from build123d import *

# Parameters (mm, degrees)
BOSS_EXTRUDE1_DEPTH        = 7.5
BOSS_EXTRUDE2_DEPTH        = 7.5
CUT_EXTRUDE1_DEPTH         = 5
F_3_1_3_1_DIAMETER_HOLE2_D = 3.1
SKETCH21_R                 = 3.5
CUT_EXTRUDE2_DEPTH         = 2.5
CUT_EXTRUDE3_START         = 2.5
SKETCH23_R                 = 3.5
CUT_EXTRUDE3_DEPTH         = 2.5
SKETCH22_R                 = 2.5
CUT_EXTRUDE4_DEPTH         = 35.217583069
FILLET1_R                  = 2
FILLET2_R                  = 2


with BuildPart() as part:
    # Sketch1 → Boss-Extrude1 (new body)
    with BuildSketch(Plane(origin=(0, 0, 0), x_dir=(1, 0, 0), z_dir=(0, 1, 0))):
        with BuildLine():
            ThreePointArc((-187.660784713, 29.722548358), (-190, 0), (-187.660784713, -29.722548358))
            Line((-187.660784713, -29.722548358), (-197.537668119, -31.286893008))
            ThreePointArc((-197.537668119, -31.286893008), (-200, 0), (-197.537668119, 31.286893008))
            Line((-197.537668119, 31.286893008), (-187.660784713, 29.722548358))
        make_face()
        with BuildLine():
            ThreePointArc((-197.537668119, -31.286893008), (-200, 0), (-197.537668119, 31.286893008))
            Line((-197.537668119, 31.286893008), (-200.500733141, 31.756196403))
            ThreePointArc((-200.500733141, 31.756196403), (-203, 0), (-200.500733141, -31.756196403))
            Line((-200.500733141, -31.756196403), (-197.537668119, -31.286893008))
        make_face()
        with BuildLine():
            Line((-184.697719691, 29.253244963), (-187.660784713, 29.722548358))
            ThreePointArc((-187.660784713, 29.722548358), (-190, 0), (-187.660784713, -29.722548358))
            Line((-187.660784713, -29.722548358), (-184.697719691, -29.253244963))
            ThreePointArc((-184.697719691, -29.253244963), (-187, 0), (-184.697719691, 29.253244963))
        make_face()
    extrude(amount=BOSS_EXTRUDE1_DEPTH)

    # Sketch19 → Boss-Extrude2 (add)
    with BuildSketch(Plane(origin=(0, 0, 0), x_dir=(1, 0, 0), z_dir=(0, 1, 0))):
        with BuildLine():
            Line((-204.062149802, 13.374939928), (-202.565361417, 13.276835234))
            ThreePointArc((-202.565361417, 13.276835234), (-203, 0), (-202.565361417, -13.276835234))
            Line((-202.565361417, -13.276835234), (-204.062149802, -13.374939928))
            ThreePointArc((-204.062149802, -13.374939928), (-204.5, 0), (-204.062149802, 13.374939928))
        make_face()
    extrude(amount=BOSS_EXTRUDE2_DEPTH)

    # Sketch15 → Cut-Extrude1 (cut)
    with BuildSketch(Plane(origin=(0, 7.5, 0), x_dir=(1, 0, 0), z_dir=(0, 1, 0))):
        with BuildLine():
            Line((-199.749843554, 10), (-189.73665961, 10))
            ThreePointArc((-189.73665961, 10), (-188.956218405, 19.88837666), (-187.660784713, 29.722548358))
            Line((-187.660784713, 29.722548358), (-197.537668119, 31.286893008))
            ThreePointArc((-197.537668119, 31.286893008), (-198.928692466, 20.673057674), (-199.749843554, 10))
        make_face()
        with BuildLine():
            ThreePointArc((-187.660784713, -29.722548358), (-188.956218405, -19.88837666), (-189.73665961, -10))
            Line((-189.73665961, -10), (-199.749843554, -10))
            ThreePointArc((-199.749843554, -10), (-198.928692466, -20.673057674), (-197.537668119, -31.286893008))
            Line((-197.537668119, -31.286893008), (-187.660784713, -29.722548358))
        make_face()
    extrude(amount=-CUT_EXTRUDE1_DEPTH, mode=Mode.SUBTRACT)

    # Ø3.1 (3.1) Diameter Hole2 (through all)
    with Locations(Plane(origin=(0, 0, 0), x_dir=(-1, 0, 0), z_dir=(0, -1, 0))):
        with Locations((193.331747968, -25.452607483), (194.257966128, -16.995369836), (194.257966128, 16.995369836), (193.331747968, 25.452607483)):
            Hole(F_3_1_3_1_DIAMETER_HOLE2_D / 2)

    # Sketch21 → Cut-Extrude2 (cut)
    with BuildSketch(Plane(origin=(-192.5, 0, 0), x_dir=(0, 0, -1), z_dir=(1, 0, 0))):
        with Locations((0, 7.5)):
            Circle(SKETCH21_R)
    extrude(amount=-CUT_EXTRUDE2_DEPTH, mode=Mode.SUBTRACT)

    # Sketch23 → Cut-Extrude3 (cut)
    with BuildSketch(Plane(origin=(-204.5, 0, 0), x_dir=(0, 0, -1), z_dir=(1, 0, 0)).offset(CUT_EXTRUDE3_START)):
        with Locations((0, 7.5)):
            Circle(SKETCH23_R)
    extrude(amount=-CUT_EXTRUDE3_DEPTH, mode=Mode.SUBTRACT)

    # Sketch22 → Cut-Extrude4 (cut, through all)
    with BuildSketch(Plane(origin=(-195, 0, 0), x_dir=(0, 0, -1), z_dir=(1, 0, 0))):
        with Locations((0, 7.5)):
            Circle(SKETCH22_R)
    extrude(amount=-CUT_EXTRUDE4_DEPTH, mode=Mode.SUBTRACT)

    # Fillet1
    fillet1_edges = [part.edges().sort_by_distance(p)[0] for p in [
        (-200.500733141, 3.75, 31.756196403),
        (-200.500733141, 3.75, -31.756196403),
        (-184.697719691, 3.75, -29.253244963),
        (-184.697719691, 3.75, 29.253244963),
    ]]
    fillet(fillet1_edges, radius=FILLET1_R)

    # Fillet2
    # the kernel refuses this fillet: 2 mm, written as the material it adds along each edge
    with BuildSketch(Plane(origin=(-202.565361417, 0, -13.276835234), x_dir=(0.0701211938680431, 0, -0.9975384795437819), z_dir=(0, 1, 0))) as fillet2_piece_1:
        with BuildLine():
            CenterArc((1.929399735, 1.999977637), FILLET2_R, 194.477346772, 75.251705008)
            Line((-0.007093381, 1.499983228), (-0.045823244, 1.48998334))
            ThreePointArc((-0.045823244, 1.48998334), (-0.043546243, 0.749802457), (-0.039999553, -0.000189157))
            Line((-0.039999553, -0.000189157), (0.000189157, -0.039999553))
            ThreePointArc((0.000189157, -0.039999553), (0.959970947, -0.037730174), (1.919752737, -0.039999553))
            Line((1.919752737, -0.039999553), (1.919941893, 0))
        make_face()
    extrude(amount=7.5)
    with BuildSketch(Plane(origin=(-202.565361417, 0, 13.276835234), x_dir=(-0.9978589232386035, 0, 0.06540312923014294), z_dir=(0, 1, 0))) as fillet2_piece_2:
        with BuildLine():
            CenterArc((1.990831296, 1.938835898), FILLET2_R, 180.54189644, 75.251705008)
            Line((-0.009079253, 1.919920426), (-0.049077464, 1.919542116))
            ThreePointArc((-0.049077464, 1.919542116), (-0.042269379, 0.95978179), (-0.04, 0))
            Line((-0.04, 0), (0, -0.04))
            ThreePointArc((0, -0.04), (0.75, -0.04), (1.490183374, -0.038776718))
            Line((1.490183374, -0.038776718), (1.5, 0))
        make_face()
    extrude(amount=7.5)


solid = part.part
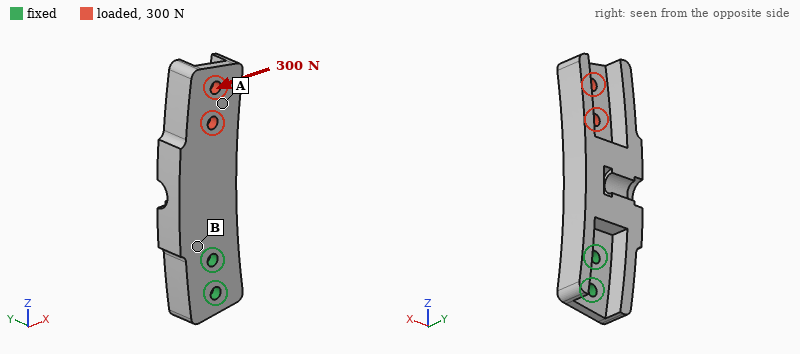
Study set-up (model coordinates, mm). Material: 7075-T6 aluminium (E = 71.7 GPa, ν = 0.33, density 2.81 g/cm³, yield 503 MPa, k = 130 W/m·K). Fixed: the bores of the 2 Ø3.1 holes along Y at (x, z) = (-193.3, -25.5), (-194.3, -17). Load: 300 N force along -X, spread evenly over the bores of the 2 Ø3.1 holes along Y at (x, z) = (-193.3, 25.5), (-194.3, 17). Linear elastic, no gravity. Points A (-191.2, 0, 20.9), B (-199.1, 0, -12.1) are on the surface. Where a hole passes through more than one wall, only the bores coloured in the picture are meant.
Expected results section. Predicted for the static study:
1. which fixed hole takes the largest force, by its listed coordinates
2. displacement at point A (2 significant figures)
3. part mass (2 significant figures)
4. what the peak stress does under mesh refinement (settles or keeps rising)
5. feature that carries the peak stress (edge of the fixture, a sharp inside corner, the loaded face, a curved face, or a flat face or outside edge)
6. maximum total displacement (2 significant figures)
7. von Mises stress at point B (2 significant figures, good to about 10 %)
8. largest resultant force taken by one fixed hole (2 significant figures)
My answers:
(-194.3, -17)
0.094 mm
15 g
keeps rising
edge of the fixture
0.12 mm
32 MPa
1.2 kN
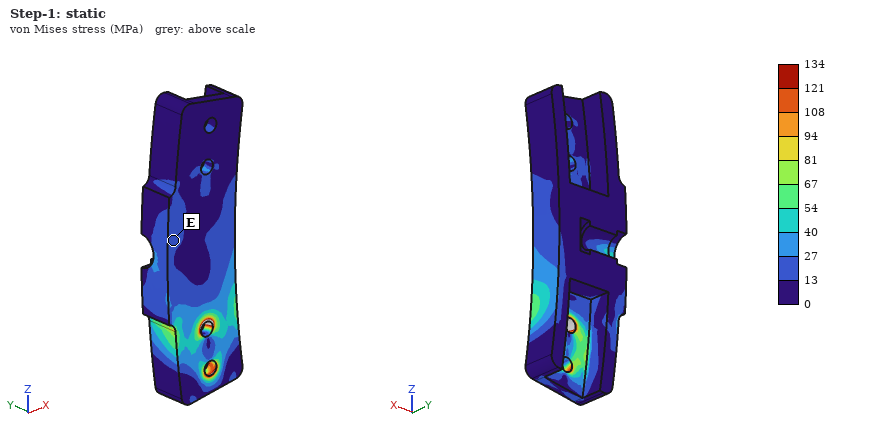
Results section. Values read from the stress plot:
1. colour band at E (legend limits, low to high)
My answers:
13 to 27 MPa
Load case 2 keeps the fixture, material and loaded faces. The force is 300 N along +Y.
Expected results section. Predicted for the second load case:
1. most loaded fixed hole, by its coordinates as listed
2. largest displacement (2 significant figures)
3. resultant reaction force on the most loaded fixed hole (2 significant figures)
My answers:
(-194.3, -17)
0.51 mm
1.2 kN
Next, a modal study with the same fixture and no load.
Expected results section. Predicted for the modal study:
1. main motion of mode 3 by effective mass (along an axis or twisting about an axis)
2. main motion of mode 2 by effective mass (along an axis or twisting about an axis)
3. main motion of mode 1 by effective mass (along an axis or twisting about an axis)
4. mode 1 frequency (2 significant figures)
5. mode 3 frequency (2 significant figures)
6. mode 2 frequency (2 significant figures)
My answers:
twisting about Z
along X
along Y
2000 Hz
5800 Hz
3900 Hz
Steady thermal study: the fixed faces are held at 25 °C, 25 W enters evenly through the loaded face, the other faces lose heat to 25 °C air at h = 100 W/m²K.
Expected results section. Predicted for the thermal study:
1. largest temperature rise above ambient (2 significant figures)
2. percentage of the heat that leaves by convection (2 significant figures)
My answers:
72 K
43 %
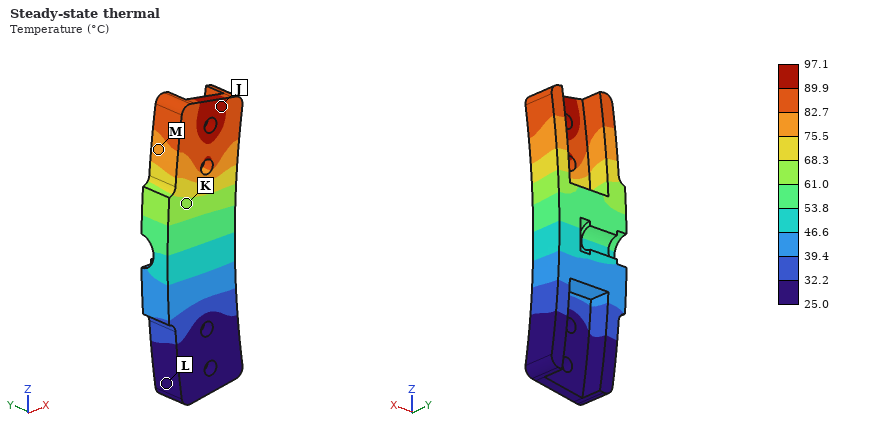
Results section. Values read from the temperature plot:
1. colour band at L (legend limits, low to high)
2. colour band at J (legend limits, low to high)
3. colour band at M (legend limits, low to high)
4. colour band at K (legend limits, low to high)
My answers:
25.0 to 32.2 °C
89.9 to 97.1 °C
75.5 to 82.7 °C
61.0 to 68.3 °C
